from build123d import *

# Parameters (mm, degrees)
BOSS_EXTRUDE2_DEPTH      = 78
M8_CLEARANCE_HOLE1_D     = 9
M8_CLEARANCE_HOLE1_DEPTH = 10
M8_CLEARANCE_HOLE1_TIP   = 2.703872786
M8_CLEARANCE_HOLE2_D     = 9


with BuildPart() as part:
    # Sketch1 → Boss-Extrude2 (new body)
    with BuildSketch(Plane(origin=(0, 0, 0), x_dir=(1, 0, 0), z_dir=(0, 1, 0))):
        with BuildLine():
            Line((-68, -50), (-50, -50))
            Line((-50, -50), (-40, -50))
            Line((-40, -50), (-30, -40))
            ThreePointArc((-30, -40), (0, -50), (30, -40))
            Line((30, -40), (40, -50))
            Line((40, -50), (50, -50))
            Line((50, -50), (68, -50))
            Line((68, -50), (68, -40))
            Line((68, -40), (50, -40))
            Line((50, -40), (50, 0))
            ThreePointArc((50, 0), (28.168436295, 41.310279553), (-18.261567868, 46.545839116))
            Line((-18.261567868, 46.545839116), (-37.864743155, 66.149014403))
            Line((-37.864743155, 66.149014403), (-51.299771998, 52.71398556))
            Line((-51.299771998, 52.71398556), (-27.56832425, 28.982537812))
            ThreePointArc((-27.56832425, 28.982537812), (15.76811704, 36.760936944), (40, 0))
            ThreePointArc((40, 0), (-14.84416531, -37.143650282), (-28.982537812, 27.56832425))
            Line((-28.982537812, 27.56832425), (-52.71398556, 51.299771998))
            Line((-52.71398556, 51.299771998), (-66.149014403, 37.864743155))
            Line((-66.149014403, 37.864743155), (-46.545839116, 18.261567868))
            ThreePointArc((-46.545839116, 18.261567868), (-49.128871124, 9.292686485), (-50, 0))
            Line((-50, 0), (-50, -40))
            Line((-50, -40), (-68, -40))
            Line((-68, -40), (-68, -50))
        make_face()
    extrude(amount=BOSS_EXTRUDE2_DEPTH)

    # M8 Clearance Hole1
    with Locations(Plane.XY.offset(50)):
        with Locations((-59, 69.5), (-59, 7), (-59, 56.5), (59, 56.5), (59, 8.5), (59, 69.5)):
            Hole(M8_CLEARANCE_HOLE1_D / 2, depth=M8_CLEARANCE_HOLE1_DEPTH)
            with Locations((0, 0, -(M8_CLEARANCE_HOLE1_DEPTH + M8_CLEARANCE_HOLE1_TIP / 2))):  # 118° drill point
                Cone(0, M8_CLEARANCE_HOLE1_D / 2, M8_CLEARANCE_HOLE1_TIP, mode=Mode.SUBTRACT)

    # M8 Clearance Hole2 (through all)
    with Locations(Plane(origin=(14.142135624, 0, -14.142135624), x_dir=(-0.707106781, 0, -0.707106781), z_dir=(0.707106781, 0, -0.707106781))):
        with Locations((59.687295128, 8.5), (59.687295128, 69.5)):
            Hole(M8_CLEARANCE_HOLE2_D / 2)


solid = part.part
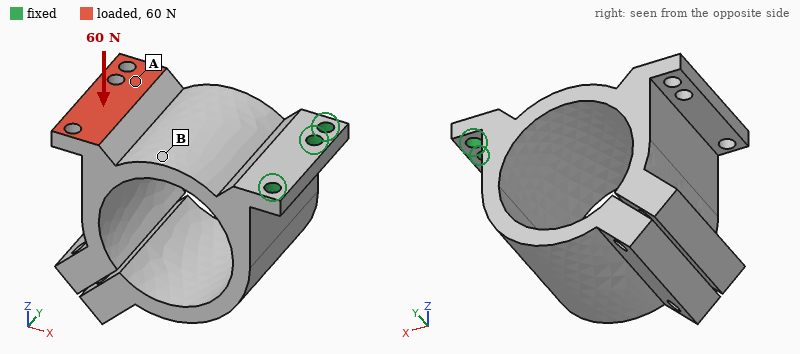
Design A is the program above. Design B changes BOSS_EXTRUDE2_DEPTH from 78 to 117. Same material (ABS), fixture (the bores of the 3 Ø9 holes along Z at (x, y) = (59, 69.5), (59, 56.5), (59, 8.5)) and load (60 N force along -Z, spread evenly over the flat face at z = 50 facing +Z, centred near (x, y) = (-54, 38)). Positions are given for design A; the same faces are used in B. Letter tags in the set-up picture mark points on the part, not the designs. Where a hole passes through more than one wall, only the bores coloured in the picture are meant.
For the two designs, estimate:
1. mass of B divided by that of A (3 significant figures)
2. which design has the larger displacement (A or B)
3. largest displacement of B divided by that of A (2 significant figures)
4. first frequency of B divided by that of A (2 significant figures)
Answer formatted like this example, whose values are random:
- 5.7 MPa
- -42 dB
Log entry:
- 1.51
- A
- 0.74
- 0.92
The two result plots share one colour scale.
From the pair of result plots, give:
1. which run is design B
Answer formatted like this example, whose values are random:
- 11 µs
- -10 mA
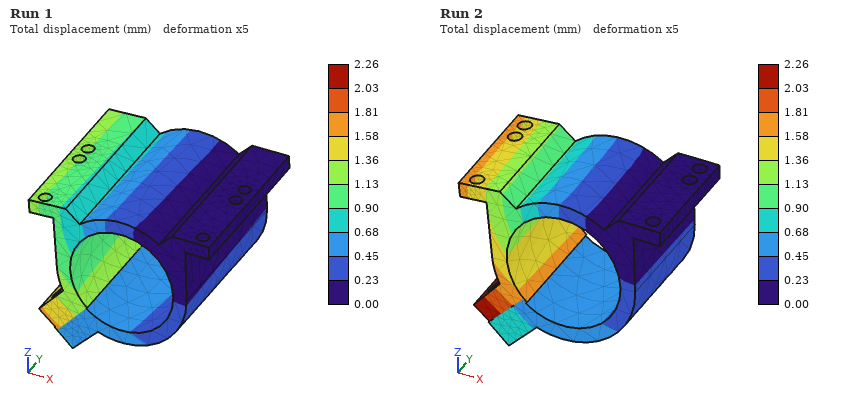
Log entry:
- Run 1
